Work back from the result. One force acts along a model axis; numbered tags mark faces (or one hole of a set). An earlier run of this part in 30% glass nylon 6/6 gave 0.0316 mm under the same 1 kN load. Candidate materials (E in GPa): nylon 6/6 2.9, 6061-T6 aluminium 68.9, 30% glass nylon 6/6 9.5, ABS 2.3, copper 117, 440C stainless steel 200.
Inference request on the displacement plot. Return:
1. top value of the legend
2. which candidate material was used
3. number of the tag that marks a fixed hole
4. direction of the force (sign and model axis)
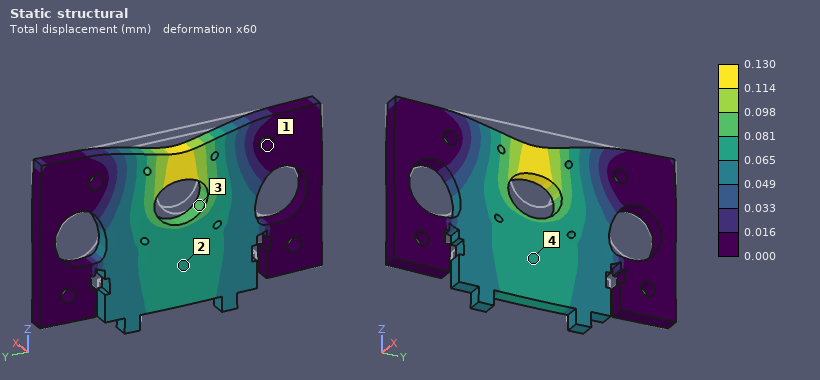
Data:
0.130 mm
ABS
1
-Z
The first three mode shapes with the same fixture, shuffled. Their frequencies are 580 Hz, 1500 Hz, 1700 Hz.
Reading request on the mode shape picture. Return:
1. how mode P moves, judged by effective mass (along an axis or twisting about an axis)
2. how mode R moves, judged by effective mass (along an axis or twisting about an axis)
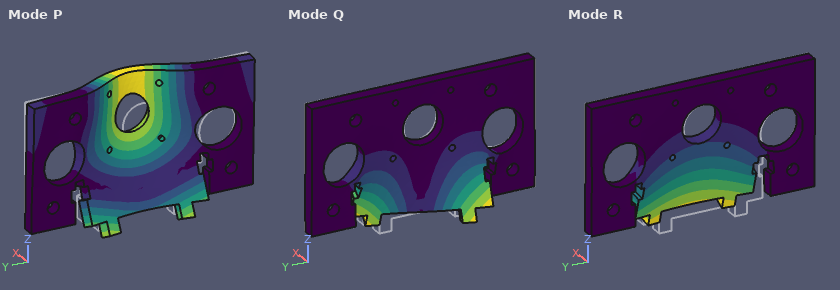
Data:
along X
along X
